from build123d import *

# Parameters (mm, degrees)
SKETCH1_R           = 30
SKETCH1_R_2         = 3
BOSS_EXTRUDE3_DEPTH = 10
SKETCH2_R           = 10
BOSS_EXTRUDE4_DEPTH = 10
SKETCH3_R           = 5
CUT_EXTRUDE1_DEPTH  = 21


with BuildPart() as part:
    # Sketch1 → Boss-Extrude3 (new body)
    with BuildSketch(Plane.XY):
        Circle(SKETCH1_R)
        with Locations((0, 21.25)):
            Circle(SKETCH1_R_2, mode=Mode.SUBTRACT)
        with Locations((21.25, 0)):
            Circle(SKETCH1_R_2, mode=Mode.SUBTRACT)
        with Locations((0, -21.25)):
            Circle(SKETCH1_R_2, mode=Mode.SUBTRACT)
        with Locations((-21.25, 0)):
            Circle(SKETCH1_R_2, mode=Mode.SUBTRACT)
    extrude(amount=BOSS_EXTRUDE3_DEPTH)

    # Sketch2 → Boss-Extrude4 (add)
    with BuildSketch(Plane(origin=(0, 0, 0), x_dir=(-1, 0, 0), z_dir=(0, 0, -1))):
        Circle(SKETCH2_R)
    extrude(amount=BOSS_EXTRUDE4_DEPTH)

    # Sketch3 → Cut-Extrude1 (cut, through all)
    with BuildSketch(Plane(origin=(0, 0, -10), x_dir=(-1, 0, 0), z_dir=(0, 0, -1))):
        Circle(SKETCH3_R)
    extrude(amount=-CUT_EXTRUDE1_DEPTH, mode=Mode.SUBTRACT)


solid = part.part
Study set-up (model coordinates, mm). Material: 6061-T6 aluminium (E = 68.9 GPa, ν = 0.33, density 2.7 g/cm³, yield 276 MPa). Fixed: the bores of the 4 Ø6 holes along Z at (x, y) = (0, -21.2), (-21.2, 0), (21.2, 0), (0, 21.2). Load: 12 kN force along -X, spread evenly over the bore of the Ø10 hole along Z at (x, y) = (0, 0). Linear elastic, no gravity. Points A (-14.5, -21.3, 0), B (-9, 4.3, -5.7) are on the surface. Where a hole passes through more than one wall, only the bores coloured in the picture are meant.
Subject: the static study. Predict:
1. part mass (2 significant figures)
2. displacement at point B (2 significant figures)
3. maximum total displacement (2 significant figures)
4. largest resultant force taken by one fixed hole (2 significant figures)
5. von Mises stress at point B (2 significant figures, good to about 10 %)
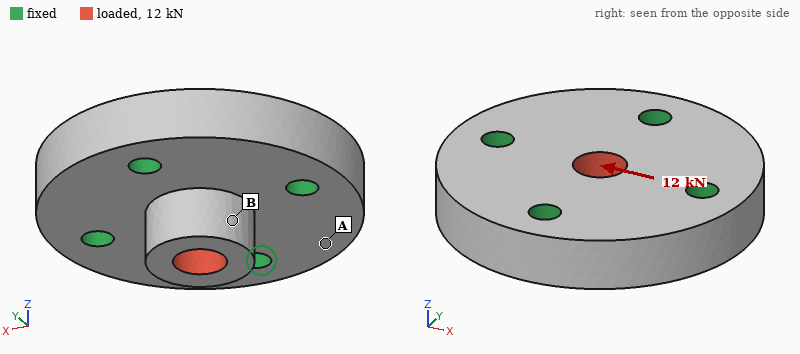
78 g
19 µm
25 µm
4.3 kN
17 MPa
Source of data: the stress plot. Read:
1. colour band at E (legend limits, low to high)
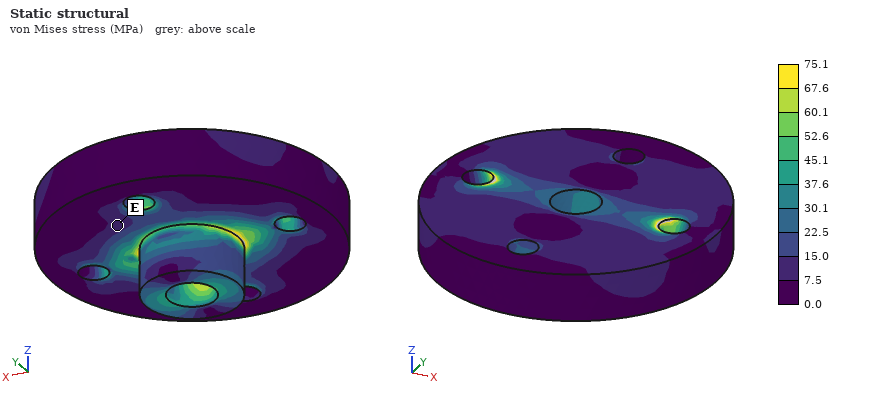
7.5 to 15.0 MPa
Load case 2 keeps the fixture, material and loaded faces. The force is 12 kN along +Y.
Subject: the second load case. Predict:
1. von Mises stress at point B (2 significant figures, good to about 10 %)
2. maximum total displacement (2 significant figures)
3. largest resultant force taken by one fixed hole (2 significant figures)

21 MPa
25 µm
4.3 kN
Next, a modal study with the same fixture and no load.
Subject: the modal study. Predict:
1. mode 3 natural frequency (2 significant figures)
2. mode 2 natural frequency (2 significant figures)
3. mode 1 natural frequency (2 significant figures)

28 kHz
28 kHz
28 kHz
